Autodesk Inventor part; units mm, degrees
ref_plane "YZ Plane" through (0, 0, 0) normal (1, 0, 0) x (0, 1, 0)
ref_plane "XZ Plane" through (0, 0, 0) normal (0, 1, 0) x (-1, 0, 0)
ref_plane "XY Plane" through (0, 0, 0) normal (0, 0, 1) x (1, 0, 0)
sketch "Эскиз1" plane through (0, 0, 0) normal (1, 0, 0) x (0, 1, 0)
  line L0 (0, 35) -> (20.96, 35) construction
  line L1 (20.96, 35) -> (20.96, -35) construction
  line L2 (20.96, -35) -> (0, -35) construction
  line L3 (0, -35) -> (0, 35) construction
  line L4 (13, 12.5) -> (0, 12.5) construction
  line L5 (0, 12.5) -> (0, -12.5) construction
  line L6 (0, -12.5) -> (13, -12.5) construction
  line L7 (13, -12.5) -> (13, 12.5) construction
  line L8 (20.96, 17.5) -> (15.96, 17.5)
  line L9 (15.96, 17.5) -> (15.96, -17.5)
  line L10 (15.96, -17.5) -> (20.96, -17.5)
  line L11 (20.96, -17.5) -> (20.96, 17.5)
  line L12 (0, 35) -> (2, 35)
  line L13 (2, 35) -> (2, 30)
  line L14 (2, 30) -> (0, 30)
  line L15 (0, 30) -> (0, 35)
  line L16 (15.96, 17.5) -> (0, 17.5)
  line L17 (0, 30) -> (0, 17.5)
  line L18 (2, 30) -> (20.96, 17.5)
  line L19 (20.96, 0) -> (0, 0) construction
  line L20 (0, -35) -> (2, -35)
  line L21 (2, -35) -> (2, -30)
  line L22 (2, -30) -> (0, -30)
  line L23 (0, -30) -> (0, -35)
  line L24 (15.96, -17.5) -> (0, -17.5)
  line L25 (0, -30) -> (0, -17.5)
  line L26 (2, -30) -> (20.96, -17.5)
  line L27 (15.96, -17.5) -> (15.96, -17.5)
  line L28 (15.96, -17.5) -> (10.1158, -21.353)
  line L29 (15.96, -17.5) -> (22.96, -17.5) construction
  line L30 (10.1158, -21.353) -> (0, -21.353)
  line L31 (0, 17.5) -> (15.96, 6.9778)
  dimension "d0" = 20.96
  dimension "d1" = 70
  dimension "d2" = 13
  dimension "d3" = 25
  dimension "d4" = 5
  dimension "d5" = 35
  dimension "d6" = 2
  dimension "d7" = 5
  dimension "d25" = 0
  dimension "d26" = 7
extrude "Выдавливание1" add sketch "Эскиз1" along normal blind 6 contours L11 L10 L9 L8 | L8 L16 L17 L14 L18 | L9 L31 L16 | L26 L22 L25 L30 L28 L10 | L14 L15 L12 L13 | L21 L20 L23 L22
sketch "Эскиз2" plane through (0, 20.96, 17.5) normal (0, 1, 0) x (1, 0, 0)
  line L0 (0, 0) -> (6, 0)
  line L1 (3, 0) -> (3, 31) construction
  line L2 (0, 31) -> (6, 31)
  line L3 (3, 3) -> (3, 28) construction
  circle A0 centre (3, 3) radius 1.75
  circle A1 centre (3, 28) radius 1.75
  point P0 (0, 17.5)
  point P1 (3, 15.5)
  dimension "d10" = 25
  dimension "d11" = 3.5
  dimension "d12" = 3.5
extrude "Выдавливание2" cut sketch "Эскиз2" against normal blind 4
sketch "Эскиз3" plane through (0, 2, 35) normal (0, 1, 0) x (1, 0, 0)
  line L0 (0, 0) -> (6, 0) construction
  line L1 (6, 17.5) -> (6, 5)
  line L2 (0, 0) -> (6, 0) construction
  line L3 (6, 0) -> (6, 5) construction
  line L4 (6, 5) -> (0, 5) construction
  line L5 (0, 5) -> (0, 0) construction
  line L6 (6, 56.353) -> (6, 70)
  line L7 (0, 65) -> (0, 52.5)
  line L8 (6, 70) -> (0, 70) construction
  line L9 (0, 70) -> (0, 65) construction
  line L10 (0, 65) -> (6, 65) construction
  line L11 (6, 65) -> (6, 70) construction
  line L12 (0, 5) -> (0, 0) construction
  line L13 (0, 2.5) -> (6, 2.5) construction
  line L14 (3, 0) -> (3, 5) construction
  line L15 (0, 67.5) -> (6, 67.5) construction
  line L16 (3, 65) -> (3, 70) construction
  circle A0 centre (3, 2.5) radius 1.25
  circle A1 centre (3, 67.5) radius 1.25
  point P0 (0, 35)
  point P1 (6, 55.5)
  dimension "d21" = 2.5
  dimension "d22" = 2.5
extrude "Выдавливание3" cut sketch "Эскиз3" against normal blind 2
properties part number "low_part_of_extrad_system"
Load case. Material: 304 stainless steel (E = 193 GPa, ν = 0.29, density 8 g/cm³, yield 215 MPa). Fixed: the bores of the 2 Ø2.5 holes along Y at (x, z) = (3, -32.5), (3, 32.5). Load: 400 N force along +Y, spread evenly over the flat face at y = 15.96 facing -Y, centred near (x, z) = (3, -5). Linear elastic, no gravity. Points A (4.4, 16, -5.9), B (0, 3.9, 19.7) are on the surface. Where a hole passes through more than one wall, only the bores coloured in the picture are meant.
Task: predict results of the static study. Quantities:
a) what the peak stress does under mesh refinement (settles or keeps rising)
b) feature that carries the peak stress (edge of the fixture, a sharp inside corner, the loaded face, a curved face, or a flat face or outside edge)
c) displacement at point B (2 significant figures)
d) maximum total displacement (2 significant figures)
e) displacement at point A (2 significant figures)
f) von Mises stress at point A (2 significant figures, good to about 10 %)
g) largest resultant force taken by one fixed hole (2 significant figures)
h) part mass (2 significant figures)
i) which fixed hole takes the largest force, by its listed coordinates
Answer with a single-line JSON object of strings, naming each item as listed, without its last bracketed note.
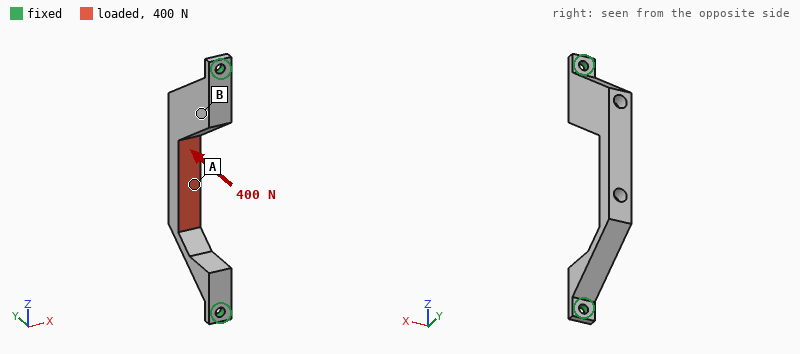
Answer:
{"what the peak stress does under mesh refinement": "keeps rising", "feature that carries the peak stress": "edge of the fixture", "displacement at point B": "5.6 µm", "maximum total displacement": "14 µm", "displacement at point A": "13 µm", "von Mises stress at point A": "30 MPa", "largest resultant force taken by one fixed hole": "310 N", "part mass": "24 g", "which fixed hole takes the largest force, by its listed coordinates": "(3, -32.5)"}
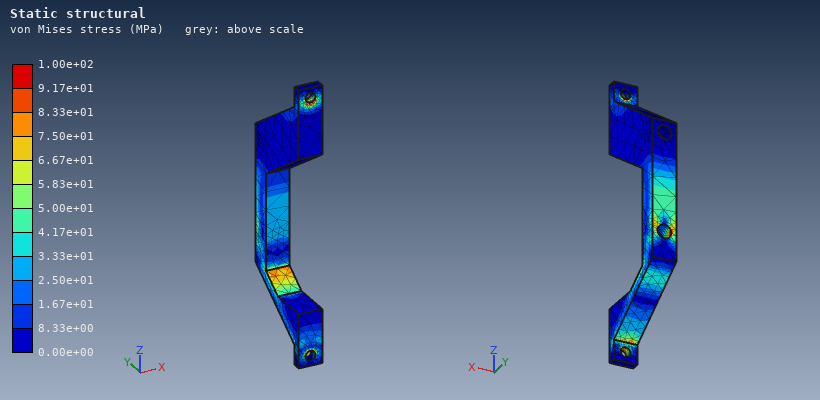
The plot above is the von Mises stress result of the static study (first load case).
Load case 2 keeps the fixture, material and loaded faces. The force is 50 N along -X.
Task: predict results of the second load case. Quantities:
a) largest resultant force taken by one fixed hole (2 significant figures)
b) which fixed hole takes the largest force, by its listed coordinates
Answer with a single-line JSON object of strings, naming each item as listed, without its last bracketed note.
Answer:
{"largest resultant force taken by one fixed hole": "29 N", "which fixed hole takes the largest force, by its listed coordinates": "(3, -32.5)"}
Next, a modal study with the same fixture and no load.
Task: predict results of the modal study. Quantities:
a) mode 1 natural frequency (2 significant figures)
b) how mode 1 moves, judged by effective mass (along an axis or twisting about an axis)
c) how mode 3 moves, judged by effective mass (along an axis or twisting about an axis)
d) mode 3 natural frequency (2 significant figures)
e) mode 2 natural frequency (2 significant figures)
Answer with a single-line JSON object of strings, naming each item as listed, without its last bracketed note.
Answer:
{"mode 1 natural frequency": "2200 Hz", "how mode 1 moves, judged by effective mass": "along X", "how mode 3 moves, judged by effective mass": "twisting about Y", "mode 3 natural frequency": "7200 Hz", "mode 2 natural frequency": "5500 Hz"}
